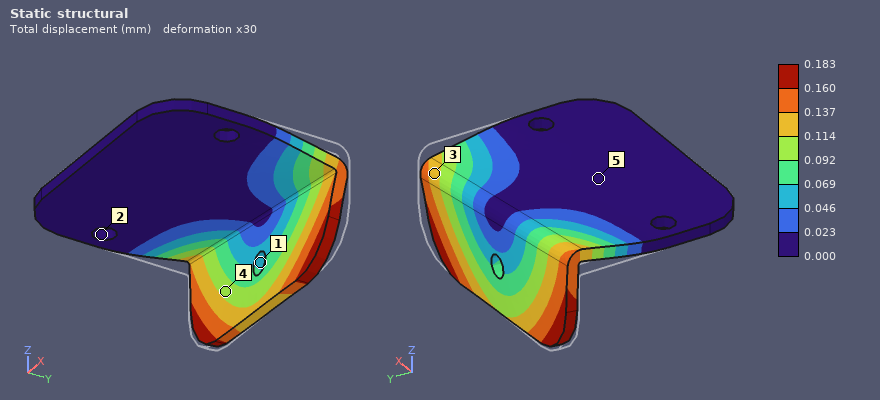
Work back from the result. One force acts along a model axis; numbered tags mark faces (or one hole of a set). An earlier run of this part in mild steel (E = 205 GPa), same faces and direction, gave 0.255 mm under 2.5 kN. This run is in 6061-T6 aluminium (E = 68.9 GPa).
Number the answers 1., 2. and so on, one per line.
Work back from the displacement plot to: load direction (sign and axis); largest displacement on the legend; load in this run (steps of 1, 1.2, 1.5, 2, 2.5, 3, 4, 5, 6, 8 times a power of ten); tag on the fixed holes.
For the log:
1. -X
2. 0.183 mm
3. 600 N
4. 2
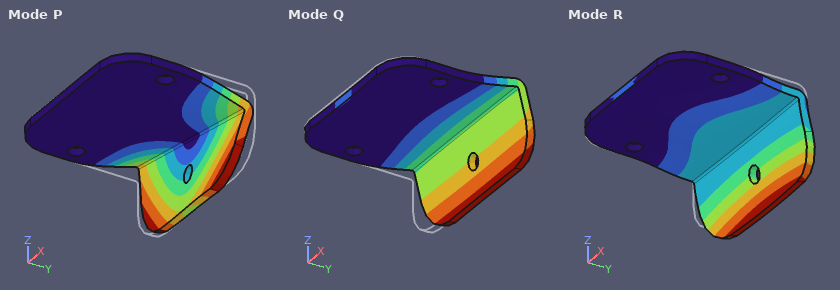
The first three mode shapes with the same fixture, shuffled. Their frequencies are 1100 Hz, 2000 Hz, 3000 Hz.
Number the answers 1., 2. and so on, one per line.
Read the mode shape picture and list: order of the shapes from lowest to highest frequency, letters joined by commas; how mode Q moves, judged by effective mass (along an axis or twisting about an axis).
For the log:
1. Q, P, R
2. along Z
